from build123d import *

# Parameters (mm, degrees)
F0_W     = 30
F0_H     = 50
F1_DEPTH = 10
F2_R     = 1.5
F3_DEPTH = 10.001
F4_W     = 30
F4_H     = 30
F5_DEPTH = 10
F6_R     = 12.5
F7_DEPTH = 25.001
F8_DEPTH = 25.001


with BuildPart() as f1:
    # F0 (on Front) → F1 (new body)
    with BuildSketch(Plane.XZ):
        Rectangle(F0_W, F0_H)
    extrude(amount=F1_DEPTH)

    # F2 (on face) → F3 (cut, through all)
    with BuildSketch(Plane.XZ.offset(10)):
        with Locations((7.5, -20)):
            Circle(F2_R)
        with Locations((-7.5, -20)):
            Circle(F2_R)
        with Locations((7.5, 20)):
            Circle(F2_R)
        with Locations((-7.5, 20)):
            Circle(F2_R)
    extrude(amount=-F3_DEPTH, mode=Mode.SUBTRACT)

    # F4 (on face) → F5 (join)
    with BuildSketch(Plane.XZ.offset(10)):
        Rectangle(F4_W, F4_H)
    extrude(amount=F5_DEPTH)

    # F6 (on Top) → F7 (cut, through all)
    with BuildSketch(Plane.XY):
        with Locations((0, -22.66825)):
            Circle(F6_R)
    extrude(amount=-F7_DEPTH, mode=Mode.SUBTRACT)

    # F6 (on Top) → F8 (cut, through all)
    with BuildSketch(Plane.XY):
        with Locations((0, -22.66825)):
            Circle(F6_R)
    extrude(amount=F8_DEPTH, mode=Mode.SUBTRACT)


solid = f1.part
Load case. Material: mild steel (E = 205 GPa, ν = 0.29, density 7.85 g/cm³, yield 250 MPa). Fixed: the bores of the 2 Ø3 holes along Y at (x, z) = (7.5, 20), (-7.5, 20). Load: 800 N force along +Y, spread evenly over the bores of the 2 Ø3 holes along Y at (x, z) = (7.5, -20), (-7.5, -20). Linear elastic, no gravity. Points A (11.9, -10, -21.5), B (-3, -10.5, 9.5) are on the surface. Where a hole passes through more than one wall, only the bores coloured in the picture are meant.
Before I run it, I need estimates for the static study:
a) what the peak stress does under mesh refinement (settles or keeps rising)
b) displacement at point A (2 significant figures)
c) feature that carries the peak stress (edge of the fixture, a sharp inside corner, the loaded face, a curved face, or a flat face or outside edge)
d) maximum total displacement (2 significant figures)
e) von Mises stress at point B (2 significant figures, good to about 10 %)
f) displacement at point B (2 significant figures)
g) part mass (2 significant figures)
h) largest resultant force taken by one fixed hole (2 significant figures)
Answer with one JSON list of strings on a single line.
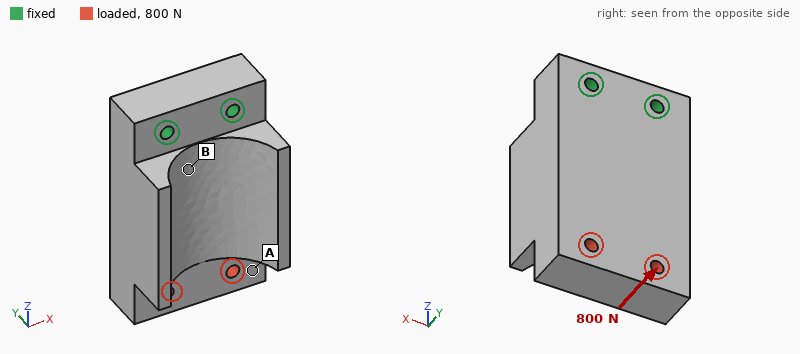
["keeps rising", "30 µm", "edge of the fixture", "34 µm", "25 MPa", "5.7 µm", "140 g", "410 N"]
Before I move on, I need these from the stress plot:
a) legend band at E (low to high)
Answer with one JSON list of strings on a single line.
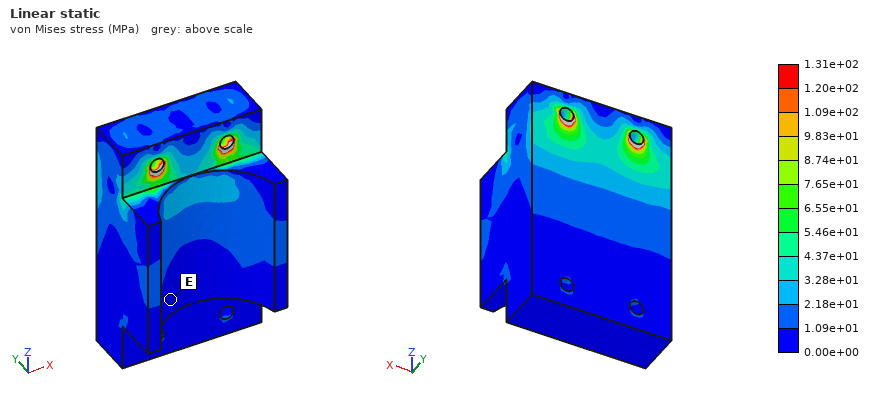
["0.00e+00 to 1.09e+01 MPa"]
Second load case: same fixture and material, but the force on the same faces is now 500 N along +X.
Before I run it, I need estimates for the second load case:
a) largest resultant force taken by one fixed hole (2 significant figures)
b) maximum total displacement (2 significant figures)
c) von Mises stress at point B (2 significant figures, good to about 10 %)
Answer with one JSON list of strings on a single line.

["1.2 kN", "5.0 µm", "4.9 MPa"]
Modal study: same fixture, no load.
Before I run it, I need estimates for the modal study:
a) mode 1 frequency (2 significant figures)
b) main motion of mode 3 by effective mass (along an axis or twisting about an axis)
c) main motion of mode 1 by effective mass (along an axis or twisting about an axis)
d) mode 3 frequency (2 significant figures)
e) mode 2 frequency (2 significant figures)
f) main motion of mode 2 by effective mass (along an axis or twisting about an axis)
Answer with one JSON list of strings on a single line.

["3800 Hz", "twisting about Z", "along Y", "9900 Hz", "7600 Hz", "along X"]
